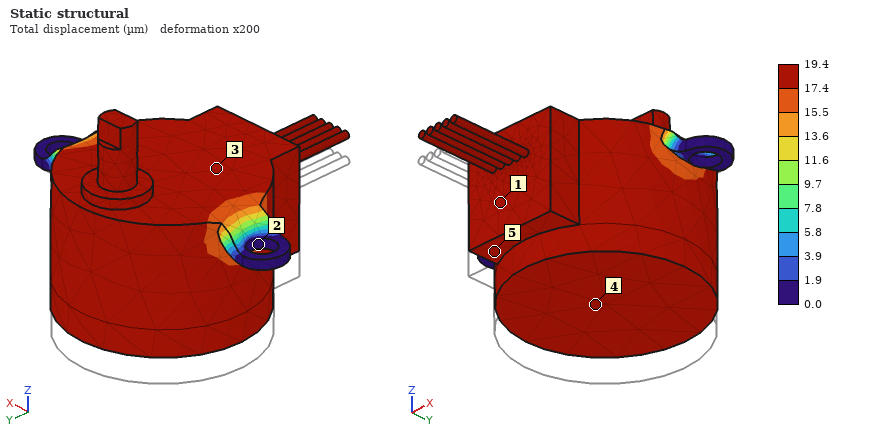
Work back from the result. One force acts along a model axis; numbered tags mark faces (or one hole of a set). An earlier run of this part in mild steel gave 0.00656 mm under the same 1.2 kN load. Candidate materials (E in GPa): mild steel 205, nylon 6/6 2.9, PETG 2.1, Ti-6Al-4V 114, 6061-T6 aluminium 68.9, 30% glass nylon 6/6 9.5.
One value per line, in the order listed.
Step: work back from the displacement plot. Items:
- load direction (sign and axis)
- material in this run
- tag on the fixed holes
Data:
+Z
6061-T6 aluminium
2
